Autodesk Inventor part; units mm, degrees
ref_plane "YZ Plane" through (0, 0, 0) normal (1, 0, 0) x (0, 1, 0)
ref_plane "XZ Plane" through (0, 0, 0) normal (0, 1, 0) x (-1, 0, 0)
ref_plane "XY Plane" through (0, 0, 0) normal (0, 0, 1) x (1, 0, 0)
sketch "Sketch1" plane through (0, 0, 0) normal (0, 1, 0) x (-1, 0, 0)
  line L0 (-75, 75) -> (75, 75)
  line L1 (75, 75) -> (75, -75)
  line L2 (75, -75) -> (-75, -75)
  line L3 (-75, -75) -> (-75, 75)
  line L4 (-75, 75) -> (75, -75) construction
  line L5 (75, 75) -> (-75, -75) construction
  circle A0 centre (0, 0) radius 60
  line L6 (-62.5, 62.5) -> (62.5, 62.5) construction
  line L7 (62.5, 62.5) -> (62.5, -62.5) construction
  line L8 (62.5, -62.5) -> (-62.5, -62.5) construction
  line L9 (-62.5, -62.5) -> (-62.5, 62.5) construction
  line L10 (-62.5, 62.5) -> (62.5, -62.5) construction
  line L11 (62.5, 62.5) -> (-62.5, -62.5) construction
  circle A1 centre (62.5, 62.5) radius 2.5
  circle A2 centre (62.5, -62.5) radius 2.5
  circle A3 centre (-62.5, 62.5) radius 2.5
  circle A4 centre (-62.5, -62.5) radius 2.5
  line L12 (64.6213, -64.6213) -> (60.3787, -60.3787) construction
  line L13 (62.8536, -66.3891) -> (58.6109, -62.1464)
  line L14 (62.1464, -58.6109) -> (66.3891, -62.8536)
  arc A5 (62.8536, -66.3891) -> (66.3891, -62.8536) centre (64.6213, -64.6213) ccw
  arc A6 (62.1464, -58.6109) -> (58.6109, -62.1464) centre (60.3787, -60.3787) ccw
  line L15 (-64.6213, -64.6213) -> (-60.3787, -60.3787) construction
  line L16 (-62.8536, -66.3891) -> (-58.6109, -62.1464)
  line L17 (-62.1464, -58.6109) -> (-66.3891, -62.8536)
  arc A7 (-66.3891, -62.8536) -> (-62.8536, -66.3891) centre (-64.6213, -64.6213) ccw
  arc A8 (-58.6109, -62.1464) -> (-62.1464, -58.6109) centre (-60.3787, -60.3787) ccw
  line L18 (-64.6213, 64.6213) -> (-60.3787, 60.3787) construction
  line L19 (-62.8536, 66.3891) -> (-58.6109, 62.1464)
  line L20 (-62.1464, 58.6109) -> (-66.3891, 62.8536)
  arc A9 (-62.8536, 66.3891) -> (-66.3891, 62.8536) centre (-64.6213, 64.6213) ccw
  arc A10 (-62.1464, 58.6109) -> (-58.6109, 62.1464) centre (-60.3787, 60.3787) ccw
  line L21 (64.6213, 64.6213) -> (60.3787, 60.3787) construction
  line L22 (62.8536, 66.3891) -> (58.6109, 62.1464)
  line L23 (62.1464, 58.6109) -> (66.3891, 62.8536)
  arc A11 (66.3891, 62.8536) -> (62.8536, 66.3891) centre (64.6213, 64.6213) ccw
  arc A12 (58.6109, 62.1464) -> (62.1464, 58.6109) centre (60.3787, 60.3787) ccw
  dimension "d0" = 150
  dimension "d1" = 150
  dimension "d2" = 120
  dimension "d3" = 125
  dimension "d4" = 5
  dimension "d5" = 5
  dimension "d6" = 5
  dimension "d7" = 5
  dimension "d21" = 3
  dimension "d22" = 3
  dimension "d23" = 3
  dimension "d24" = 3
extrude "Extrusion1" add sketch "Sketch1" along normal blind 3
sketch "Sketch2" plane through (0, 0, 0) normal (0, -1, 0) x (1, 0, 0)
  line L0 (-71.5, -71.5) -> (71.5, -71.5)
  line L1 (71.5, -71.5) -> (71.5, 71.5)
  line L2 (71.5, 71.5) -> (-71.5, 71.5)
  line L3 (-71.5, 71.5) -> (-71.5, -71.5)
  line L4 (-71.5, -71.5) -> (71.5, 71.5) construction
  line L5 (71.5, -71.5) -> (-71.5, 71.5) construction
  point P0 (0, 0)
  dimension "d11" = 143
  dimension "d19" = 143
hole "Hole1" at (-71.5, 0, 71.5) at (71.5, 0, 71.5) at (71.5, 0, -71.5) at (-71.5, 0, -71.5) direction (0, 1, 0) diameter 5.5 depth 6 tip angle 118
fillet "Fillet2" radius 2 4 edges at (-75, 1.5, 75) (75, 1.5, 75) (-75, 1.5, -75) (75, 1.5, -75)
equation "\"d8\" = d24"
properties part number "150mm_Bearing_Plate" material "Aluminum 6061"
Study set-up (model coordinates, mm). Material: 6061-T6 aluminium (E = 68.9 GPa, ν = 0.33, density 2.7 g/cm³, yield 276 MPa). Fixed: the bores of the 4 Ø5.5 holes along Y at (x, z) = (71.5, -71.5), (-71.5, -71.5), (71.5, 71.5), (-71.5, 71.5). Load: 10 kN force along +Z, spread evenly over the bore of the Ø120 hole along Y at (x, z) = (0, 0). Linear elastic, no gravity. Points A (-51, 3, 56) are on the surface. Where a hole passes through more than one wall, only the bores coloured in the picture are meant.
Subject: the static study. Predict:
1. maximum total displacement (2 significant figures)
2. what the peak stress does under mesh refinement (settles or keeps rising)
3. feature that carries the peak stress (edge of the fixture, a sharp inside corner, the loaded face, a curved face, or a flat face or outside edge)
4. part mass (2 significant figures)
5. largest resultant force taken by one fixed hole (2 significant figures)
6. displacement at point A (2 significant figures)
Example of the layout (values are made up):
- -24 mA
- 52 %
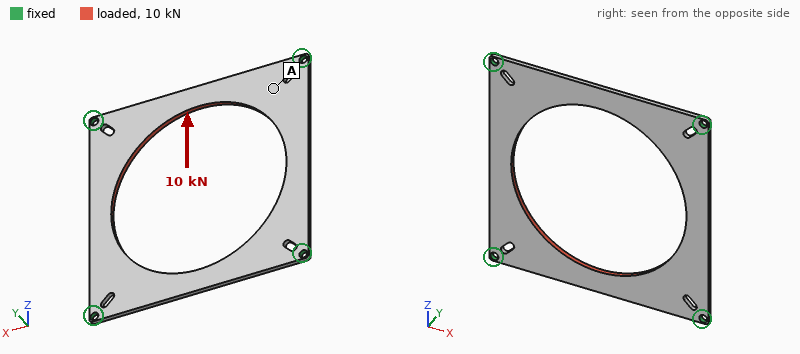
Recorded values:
- 0.19 mm
- keeps rising
- edge of the fixture
- 88 g
- 2.7 kN
- 0.067 mm
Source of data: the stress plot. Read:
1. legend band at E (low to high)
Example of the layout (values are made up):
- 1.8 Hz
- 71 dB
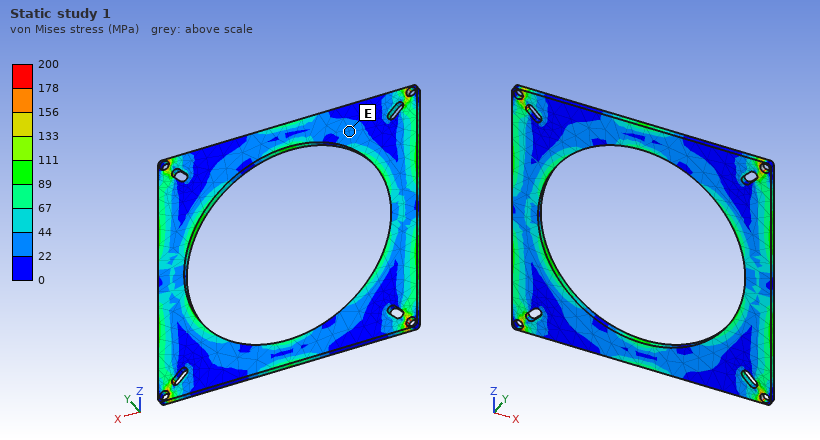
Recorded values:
- 22 to 44 MPa
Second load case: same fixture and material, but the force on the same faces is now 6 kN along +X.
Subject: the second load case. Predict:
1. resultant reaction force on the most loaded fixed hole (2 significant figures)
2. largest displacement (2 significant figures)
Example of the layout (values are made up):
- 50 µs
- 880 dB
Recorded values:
- 1.6 kN
- 0.12 mm
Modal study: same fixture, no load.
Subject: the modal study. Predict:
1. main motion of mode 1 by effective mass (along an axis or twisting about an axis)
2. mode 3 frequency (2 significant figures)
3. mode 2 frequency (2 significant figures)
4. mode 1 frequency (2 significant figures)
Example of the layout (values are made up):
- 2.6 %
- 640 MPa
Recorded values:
- along Y
- 800 Hz
- 800 Hz
- 670 Hz
